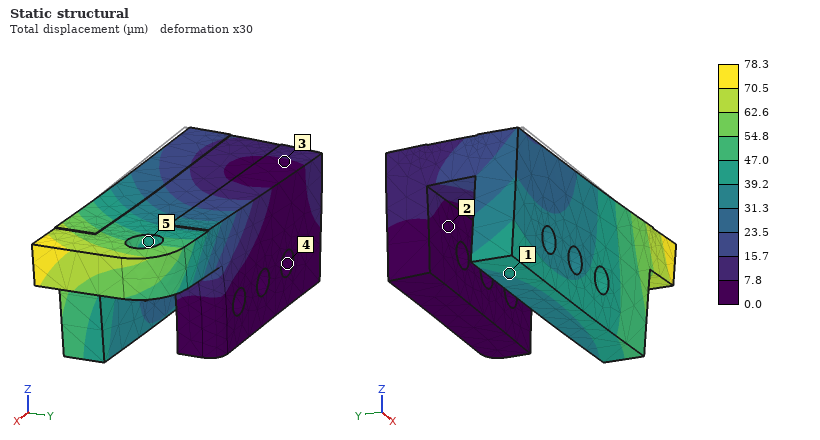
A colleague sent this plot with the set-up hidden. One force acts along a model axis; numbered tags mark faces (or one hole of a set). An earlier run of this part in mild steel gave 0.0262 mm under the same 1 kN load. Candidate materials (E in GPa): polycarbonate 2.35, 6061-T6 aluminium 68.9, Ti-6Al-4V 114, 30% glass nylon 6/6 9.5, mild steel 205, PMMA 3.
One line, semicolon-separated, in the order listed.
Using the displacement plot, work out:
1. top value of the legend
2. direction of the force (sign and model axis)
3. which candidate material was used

78.3 µm; -Y; 6061-T6 aluminium
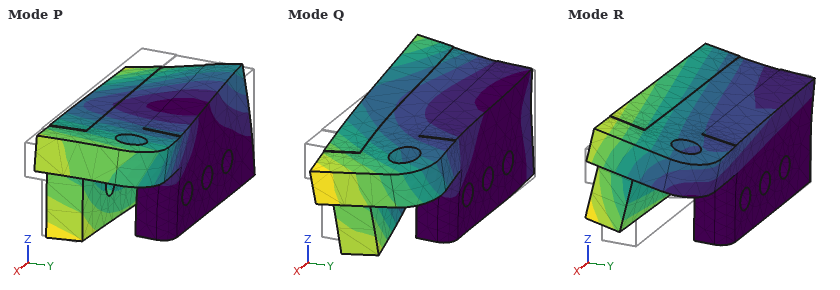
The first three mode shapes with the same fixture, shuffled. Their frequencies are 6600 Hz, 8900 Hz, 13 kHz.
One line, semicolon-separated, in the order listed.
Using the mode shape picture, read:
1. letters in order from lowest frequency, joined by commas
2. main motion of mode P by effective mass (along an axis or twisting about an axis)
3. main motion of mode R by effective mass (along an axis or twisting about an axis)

R, P, Q; along X; along Z
